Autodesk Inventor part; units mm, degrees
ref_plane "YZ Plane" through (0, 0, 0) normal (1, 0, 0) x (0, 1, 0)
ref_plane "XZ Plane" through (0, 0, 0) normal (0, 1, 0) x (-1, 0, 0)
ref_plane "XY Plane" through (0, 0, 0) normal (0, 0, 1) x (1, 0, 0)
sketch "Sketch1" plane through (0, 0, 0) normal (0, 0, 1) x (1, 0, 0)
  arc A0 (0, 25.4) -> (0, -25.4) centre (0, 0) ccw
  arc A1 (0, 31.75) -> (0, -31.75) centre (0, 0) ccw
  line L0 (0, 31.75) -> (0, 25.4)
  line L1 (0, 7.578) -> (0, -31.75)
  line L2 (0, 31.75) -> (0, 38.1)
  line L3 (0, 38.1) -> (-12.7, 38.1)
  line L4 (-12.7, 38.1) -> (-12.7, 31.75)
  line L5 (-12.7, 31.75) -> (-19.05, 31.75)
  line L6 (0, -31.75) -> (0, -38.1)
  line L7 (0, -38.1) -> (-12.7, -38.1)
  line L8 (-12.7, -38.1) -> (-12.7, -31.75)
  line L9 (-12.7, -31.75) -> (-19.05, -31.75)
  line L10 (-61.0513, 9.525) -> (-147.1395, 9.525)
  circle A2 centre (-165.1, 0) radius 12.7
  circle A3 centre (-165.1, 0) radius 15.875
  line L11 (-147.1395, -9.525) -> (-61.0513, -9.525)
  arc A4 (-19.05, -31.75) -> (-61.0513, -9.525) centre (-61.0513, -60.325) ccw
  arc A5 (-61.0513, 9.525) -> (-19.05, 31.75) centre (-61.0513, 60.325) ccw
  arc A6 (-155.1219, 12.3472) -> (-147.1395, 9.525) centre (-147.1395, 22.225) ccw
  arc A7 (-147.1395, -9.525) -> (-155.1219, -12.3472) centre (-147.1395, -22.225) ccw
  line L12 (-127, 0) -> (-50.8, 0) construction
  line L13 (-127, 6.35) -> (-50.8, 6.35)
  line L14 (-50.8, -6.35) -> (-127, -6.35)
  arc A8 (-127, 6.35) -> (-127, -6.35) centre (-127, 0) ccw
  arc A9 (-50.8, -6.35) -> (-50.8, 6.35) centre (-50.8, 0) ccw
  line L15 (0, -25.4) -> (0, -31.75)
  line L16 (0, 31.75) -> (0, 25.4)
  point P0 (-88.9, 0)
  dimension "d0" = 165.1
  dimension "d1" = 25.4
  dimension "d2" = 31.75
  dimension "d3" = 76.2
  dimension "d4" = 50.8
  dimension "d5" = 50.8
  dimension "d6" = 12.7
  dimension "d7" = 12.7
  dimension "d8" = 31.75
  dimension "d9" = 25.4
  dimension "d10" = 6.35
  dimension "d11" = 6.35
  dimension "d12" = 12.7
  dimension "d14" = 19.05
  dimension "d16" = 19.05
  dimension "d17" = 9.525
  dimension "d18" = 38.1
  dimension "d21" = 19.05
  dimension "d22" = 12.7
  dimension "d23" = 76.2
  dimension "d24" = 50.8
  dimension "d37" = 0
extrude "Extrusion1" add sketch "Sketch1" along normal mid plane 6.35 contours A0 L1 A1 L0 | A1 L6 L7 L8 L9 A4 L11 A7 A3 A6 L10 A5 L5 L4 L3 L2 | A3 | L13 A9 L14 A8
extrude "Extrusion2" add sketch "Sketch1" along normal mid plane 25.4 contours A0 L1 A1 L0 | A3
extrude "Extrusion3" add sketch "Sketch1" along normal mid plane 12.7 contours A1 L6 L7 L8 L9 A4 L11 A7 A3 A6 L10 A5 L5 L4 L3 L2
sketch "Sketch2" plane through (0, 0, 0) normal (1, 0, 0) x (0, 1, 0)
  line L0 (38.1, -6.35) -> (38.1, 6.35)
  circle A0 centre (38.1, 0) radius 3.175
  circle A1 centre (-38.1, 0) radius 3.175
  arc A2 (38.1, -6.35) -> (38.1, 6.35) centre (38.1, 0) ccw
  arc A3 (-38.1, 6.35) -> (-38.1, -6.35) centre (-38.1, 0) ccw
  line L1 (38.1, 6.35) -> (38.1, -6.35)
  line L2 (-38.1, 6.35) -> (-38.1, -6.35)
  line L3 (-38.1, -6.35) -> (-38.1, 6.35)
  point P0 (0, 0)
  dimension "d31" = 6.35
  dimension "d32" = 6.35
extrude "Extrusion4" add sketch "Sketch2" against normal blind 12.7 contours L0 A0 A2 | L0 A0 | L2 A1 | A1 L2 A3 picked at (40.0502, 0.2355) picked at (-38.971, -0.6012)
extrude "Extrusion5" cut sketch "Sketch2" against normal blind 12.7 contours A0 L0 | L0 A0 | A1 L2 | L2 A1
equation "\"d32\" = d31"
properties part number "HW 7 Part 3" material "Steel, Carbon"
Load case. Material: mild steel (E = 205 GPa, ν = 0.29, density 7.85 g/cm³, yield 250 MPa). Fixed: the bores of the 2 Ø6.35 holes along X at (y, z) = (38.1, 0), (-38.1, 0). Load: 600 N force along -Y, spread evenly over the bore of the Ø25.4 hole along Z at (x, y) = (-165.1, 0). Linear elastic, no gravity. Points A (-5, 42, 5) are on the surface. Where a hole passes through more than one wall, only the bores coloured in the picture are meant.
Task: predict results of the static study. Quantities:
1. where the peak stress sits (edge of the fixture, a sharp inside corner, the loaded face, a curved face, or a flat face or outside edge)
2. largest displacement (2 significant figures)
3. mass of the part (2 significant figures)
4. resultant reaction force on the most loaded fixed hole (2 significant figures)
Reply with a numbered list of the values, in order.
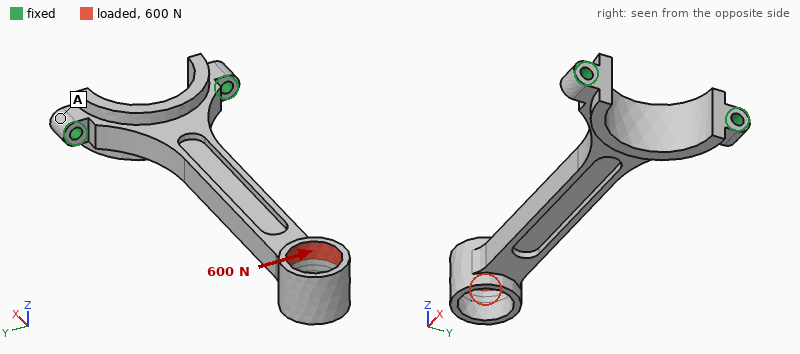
1. a curved face
2. 0.45 mm
3. 410 g
4. 1.8 kN
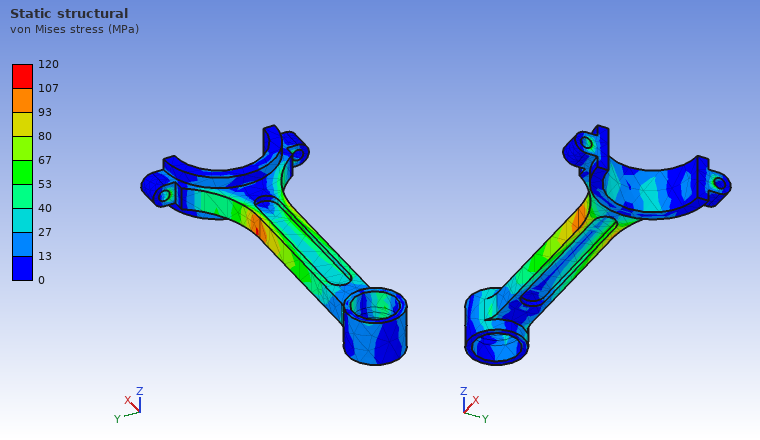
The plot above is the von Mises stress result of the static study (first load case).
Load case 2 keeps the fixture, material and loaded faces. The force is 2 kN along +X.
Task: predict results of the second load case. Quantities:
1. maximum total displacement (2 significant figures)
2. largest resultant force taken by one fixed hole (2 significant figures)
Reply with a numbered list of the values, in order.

1. 0.60 mm
2. 1.3 kN
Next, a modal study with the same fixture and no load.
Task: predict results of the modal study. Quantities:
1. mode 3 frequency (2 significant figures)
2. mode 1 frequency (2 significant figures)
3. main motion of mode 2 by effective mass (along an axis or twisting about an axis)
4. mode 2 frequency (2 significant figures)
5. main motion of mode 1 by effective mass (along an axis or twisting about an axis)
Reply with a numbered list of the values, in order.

1. 1800 Hz
2. 310 Hz
3. along Y
4. 710 Hz
5. along Z
